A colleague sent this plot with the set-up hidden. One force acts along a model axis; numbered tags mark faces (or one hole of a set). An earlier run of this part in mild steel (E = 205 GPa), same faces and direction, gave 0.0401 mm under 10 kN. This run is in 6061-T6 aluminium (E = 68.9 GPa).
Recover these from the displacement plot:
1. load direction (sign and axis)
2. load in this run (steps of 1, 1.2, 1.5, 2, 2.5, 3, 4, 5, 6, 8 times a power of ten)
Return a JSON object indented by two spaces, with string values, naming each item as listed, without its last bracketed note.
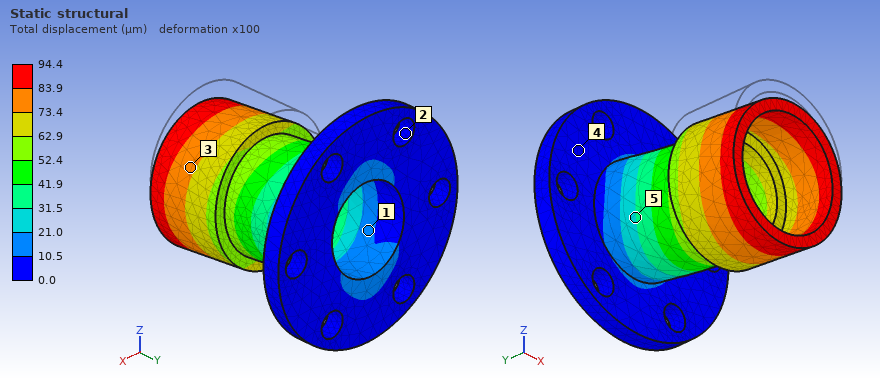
{
  "load direction": "-Z",
  "load in this run": "8 kN"
}
